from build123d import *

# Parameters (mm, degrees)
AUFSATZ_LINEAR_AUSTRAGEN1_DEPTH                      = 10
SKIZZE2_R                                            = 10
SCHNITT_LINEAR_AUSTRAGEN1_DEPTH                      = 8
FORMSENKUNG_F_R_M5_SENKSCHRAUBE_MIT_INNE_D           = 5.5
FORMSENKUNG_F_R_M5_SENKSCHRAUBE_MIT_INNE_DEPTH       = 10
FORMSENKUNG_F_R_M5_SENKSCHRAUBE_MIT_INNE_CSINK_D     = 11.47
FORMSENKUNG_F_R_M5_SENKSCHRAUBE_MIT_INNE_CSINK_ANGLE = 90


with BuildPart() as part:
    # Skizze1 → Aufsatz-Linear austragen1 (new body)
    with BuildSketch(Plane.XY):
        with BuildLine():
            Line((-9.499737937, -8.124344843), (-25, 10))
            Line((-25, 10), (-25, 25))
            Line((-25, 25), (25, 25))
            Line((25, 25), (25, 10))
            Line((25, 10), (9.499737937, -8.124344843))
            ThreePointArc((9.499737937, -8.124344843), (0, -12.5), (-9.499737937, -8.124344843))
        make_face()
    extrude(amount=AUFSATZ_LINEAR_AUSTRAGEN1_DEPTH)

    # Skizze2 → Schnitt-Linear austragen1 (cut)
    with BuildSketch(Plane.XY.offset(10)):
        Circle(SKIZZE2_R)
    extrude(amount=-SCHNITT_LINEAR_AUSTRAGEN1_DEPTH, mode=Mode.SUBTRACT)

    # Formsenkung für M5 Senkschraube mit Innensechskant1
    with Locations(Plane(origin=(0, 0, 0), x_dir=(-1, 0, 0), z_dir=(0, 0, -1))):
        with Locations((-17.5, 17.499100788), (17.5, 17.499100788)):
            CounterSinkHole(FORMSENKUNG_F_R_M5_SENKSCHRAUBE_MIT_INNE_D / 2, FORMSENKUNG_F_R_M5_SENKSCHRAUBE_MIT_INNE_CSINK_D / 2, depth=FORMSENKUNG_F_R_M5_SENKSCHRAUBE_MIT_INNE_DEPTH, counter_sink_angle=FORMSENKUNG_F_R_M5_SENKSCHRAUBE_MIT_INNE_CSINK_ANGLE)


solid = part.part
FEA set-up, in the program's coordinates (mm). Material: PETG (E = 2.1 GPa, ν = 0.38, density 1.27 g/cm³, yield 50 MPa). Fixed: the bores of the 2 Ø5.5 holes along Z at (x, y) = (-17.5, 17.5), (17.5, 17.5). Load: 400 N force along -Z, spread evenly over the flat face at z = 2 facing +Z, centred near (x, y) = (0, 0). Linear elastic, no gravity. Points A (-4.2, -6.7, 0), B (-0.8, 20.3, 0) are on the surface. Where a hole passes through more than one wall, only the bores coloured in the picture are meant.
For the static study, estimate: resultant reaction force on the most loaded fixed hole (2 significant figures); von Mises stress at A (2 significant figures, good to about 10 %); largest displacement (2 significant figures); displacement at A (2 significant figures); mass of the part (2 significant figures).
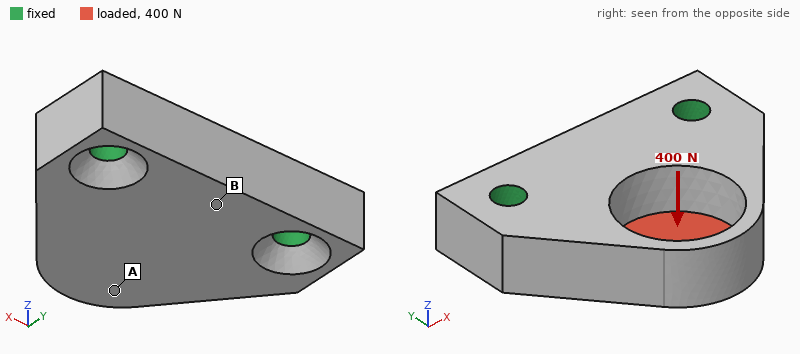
210 N
11 MPa
0.63 mm
0.53 mm
14 g
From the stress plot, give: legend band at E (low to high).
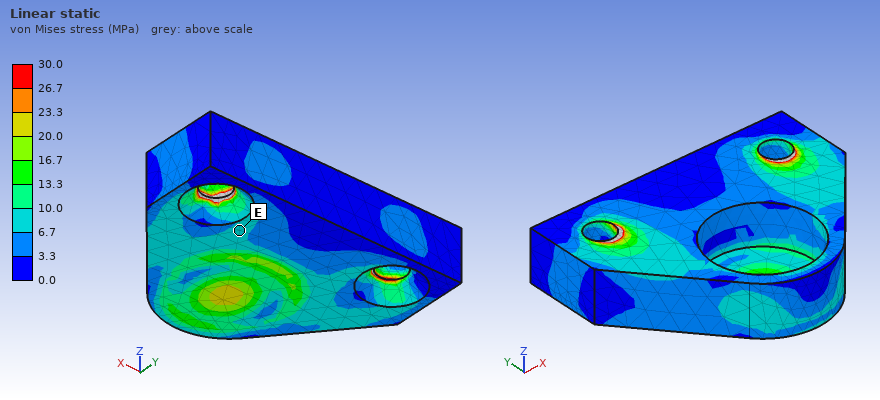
6.7 to 10.0 MPa
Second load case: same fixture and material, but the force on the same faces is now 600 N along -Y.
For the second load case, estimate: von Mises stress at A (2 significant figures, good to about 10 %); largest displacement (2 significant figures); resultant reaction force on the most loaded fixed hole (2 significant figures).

4.9 MPa
0.21 mm
310 N
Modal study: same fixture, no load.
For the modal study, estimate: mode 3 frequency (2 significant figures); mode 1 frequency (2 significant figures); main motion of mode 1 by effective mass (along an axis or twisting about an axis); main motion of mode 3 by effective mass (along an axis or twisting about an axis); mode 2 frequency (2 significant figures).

7000 Hz
2600 Hz
along Z
along Z
5000 Hz
